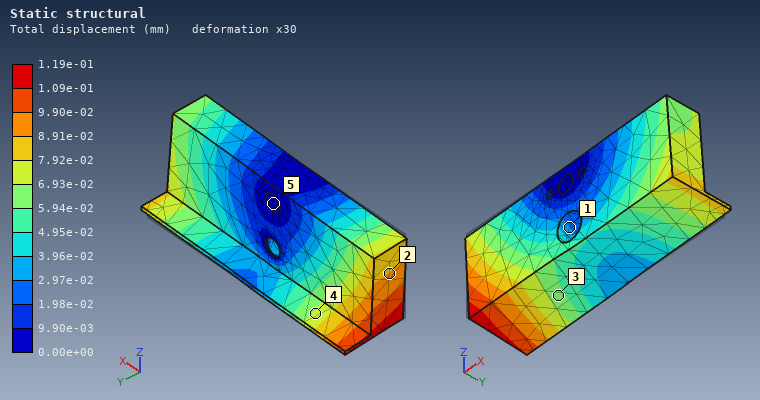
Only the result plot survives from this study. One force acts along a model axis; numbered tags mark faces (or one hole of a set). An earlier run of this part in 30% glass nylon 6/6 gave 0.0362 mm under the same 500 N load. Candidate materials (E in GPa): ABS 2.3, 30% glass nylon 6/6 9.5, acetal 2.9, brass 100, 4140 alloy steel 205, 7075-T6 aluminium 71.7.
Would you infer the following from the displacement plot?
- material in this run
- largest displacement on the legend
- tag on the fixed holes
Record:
acetal
1.19e-01 mm
5
